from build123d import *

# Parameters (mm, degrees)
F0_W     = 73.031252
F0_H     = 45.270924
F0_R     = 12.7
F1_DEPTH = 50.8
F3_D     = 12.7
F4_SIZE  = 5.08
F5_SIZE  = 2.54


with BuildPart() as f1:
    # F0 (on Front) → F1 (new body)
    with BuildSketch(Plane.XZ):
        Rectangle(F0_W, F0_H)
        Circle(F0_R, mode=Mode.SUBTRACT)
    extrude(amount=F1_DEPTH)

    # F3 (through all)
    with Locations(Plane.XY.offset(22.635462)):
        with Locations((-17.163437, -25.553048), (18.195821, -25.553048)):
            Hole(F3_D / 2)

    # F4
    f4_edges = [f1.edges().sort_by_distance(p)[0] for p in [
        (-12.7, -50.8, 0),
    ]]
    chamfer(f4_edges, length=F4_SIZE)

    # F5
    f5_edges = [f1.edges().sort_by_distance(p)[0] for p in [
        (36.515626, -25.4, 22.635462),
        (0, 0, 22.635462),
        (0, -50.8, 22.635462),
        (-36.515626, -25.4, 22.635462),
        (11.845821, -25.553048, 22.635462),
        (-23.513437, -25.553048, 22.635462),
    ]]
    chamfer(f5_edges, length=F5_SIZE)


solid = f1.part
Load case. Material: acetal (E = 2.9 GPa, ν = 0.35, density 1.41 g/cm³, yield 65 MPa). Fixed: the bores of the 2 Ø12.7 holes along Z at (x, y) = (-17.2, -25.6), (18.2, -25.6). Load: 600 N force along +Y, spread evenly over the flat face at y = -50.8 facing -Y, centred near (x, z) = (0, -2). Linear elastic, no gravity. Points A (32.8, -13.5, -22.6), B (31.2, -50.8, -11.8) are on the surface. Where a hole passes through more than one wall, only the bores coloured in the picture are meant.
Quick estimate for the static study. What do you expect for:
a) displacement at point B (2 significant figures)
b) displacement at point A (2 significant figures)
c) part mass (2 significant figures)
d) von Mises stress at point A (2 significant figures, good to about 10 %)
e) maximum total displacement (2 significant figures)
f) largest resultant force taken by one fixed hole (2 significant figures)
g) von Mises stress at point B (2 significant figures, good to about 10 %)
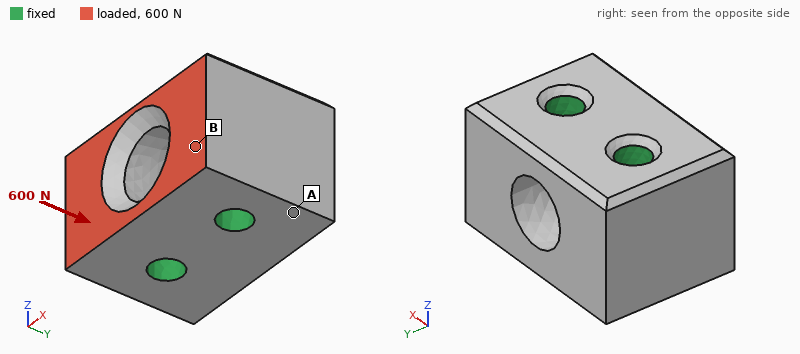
3.7 µm
0.95 µm
180 g
0.087 MPa
4.7 µm
300 N
0.29 MPa
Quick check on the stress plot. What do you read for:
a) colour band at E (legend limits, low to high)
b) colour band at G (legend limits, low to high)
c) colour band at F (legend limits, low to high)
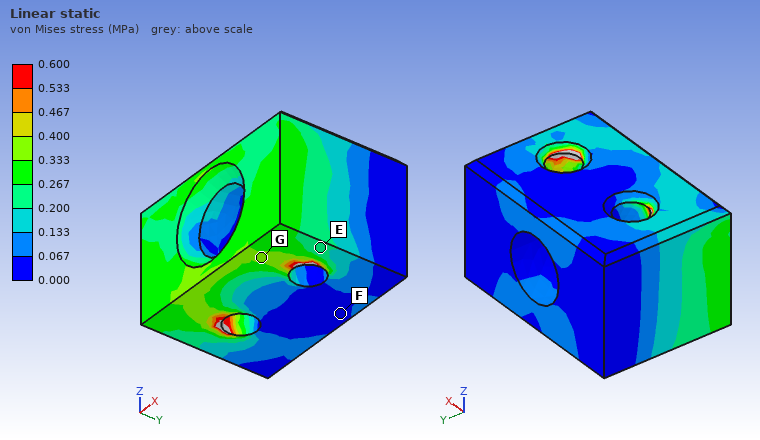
0.200 to 0.267 MPa
0.333 to 0.400 MPa
0.000 to 0.067 MPa
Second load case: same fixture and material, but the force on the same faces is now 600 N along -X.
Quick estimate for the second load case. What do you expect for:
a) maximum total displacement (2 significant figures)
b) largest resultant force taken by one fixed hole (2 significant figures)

14 µm
370 N
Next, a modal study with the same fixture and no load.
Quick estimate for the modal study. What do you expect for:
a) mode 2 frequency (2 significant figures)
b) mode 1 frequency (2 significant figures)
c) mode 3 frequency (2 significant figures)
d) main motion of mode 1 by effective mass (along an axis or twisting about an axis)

6800 Hz
5800 Hz
6900 Hz
twisting about Z
